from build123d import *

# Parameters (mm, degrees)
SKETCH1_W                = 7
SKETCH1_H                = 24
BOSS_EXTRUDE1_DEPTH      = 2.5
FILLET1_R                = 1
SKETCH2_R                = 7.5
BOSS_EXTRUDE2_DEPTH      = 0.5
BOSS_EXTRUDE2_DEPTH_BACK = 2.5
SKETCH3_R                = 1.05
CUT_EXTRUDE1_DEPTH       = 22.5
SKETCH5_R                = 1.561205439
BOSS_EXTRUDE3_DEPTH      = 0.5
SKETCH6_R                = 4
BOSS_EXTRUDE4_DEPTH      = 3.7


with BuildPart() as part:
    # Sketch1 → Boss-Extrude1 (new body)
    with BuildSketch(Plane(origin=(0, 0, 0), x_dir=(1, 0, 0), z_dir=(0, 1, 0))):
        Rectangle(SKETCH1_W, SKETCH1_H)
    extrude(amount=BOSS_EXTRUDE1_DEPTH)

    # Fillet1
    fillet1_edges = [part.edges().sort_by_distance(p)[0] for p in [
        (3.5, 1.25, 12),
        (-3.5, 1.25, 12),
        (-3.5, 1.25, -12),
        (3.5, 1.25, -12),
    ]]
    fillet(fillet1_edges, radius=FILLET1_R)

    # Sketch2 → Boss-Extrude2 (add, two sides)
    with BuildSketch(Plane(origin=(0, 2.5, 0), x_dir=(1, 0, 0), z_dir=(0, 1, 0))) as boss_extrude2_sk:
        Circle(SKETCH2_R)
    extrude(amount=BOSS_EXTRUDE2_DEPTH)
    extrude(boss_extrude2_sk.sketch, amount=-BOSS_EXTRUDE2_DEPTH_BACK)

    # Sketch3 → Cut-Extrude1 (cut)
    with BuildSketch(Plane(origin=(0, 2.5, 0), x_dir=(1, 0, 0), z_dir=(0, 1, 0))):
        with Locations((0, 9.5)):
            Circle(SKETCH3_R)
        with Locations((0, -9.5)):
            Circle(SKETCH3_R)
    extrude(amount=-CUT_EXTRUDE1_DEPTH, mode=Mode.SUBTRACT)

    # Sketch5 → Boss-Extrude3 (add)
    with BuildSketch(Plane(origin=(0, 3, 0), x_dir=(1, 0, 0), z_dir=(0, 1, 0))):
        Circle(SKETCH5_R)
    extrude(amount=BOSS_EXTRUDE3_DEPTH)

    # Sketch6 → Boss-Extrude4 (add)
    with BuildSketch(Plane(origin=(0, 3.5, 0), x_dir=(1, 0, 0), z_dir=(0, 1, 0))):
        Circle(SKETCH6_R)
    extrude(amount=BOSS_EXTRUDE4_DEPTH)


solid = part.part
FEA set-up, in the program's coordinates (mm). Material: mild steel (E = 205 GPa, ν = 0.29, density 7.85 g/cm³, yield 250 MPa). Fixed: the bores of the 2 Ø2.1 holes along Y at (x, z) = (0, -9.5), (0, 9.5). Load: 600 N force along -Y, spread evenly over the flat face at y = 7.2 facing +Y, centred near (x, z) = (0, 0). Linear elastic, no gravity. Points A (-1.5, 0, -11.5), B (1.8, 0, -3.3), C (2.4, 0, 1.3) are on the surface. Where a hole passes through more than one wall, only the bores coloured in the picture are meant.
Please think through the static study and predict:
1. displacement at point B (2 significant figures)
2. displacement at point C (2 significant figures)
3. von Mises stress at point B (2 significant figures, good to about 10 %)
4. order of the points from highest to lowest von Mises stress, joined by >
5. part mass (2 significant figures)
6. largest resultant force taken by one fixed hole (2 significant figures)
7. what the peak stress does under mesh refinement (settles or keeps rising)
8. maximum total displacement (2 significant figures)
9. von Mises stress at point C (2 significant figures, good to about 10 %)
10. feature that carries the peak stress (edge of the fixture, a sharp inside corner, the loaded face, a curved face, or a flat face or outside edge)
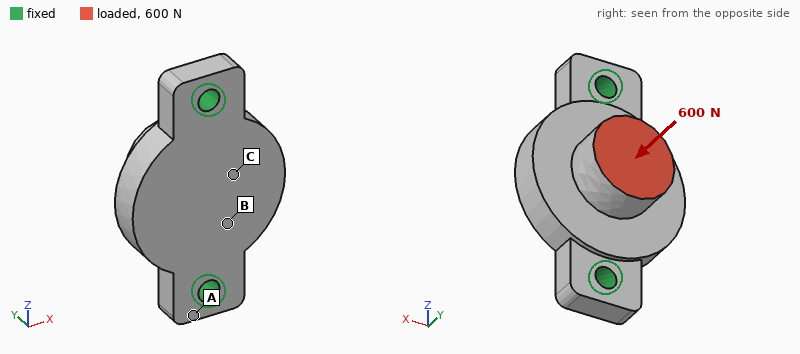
5.1 µm
6.1 µm
39 MPa
C > B > A
6.8 g
320 N
keeps rising
7.7 µm
61 MPa
edge of the fixture
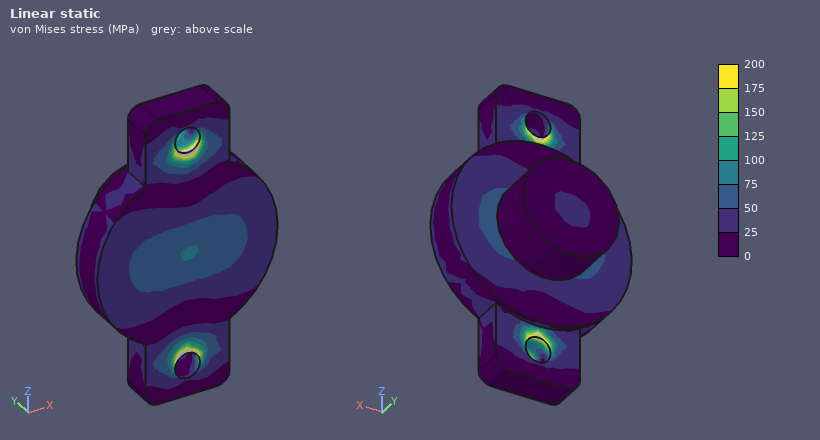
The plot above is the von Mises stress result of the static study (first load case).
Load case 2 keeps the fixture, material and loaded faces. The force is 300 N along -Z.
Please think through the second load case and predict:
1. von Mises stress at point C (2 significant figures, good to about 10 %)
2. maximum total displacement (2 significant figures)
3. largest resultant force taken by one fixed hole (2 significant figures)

27 MPa
17 µm
190 N
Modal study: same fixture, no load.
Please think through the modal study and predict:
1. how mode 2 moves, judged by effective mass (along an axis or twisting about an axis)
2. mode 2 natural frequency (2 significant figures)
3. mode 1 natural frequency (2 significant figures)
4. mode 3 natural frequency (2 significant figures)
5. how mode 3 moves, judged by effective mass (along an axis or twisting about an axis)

along Y
23 kHz
17 kHz
26 kHz
along Z
